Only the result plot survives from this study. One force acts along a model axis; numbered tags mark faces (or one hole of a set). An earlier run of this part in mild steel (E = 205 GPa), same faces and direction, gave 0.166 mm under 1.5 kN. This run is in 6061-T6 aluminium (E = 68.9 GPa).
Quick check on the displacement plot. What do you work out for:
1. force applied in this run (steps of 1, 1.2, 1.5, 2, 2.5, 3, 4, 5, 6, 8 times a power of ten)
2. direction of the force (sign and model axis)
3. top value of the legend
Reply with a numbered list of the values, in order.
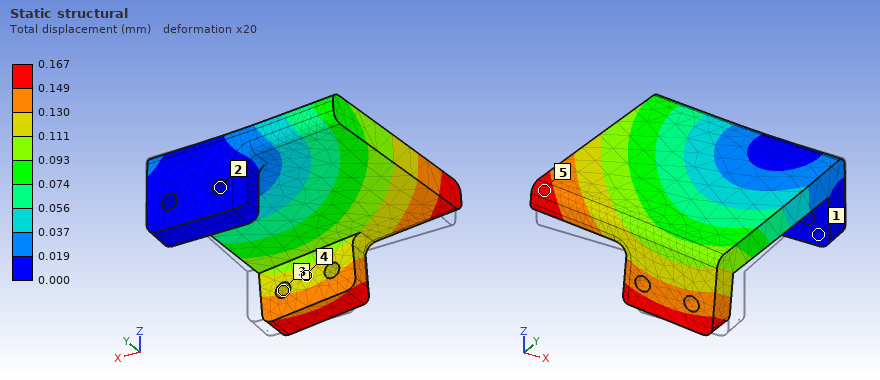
1. 500 N
2. -X
3. 0.167 mm
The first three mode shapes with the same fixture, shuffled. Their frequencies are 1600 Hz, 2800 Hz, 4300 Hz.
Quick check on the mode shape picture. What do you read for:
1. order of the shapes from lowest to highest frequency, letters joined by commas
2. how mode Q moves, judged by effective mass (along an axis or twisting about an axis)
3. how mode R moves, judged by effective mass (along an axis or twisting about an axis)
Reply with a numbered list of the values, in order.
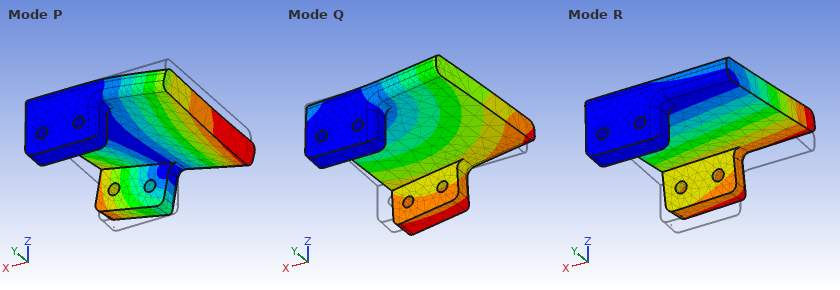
1. R, Q, P
2. along X
3. along Z
